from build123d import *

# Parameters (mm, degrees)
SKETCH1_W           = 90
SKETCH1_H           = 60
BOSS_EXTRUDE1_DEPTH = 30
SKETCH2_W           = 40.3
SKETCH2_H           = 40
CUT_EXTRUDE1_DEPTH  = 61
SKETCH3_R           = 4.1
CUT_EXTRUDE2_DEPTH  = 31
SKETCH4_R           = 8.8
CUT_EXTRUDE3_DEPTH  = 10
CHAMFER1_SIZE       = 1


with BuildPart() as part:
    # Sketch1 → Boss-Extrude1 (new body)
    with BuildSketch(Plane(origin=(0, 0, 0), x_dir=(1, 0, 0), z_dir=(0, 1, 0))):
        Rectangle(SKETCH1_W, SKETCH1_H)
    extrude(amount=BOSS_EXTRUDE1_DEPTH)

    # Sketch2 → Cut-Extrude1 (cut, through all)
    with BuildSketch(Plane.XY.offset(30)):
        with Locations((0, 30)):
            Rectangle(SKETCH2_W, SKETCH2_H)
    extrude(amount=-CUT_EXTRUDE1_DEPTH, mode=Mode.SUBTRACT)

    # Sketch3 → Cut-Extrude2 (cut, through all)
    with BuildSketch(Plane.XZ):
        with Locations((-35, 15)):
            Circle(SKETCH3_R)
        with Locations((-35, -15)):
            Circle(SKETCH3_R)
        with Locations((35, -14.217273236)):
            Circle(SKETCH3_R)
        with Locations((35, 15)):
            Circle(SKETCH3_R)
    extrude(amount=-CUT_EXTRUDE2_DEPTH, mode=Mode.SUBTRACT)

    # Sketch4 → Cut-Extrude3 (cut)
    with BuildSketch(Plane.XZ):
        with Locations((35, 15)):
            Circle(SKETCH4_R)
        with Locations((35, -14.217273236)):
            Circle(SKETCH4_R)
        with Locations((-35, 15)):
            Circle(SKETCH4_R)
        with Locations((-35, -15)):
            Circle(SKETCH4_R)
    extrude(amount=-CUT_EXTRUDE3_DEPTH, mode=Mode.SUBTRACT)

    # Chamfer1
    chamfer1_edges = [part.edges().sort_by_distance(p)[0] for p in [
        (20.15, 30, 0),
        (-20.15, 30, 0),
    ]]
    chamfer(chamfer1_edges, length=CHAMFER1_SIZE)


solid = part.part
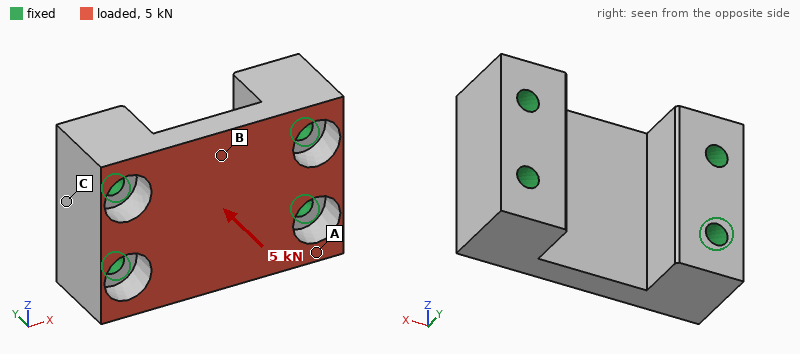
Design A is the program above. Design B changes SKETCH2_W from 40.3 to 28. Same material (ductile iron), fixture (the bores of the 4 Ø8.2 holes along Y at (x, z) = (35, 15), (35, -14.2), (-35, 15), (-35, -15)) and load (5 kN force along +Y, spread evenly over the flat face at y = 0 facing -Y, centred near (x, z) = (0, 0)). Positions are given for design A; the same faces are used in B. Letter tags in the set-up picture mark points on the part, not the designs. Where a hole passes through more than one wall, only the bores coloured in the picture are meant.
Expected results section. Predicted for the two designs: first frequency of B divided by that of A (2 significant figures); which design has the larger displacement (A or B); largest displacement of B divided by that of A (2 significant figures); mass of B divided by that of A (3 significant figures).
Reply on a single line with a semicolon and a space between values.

1.1; A; 0.58; 1.15
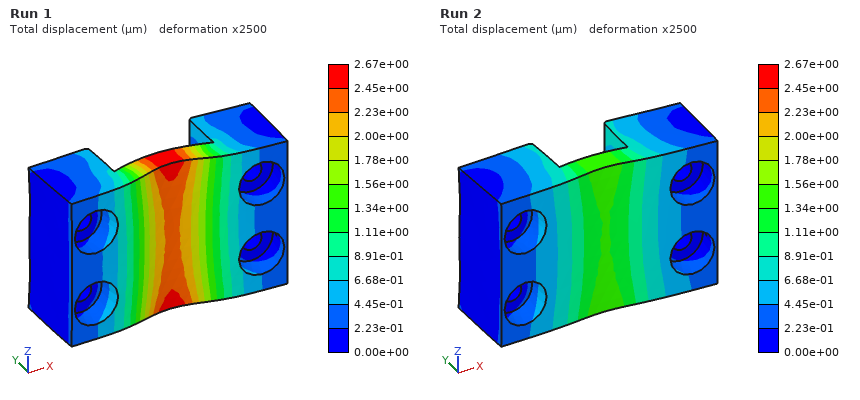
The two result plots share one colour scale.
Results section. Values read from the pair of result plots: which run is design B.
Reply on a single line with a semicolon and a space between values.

Run 2
